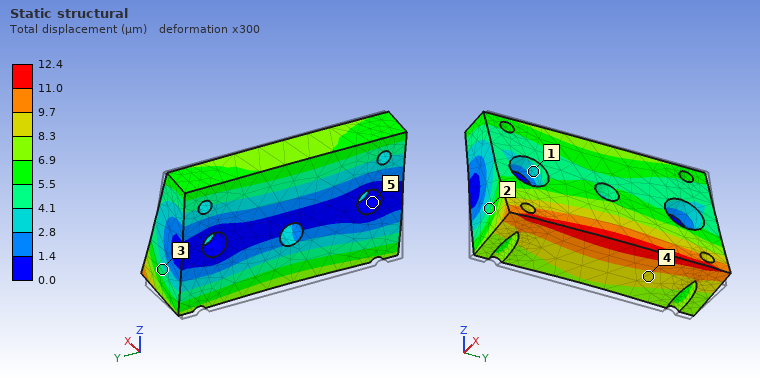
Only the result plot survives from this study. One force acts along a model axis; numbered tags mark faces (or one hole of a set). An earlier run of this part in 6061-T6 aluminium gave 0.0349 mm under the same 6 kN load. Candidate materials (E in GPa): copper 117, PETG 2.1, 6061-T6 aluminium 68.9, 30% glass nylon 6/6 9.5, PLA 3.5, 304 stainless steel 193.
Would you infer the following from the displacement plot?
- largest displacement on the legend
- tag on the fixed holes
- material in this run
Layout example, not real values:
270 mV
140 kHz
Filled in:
12.4 µm
5
304 stainless steel
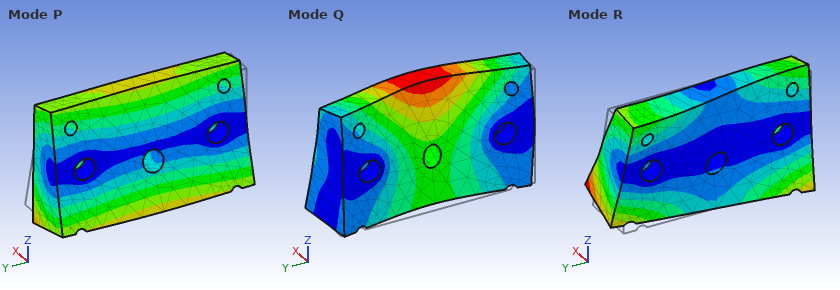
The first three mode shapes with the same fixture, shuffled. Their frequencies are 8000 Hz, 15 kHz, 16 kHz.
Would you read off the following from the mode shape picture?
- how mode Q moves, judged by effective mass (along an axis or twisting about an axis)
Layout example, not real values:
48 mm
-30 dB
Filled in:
along X
